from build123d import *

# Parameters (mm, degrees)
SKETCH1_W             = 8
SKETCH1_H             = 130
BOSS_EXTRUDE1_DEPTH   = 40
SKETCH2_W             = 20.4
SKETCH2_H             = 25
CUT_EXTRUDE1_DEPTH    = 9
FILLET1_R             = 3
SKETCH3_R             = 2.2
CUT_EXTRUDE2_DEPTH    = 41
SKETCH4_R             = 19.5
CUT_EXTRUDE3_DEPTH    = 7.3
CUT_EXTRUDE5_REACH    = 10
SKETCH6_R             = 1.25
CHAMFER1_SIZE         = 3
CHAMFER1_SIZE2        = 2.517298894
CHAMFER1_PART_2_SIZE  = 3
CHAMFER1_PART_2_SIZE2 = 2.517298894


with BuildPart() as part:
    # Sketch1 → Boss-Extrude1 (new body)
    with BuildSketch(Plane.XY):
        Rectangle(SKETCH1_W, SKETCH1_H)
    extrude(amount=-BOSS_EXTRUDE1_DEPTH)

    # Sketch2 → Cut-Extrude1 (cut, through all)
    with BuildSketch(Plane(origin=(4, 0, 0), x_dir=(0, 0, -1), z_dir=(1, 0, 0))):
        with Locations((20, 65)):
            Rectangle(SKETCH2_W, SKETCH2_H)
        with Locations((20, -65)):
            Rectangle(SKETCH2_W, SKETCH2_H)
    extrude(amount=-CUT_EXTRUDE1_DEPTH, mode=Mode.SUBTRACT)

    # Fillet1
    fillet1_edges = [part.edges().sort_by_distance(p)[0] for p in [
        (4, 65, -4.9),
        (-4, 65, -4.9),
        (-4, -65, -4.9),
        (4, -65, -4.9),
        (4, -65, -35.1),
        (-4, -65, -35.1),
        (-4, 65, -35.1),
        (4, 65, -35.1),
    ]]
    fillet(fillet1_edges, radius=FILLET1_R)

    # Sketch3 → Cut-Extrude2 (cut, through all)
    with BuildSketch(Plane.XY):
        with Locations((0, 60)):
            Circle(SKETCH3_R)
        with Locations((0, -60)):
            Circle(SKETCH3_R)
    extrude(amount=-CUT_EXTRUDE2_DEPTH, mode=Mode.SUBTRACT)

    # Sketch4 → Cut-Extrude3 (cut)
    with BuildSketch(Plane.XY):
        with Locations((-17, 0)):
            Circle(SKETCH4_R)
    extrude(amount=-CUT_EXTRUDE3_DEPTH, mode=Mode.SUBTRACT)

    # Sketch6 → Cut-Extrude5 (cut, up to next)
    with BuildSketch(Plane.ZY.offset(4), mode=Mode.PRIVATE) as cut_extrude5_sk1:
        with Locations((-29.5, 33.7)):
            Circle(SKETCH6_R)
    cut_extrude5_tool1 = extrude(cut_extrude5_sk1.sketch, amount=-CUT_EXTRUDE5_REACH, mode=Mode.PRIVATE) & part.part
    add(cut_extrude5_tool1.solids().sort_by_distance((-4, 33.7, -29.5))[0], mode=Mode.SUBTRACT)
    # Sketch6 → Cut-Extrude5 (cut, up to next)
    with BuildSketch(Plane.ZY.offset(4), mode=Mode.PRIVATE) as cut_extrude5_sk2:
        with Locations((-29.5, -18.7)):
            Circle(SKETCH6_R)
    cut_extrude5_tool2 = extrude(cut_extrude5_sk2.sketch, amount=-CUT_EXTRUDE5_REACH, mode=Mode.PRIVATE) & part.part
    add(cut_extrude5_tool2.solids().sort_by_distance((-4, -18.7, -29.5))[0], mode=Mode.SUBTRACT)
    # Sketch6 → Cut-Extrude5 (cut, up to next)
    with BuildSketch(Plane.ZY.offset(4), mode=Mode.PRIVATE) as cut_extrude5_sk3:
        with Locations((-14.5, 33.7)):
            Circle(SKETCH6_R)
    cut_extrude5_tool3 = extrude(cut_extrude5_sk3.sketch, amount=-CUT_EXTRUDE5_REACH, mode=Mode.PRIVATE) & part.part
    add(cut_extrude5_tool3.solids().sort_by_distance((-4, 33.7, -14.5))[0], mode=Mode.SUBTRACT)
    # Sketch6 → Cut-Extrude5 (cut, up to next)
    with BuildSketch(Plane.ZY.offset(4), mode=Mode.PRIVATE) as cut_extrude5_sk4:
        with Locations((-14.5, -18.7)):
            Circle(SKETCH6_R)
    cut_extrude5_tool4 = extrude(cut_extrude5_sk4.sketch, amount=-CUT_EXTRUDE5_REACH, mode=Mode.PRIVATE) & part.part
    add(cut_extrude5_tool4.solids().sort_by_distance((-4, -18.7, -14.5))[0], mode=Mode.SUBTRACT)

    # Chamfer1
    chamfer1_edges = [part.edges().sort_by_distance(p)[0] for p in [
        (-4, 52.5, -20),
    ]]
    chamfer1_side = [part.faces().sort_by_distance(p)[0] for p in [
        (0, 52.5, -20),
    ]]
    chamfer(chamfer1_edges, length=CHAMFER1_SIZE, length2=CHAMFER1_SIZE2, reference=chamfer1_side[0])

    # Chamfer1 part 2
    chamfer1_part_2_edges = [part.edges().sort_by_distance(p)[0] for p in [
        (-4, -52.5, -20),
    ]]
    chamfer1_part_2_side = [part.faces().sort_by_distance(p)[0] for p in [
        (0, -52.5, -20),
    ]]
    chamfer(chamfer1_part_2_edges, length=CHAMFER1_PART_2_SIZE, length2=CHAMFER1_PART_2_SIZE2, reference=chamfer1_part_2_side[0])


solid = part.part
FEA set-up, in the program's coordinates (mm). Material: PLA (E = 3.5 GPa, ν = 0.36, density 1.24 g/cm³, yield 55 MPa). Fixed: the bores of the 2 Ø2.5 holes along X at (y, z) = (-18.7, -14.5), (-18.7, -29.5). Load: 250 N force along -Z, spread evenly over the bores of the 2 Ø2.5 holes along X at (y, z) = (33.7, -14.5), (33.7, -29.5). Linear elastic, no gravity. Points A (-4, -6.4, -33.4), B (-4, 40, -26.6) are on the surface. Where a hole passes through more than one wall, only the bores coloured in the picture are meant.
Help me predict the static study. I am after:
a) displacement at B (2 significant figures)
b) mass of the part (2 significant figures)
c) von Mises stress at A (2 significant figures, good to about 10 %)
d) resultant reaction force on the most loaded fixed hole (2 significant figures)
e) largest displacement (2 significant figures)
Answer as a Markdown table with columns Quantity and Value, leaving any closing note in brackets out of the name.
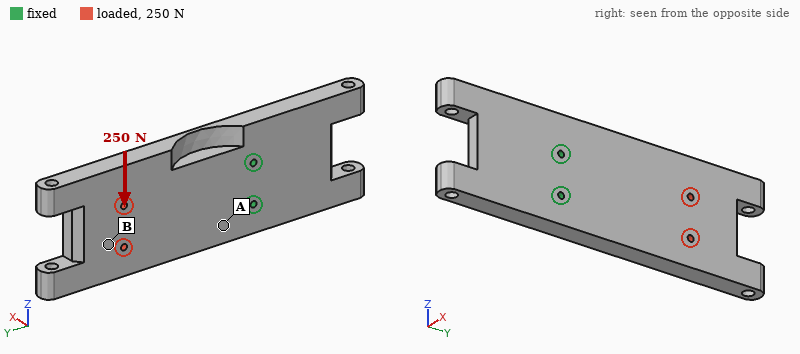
| Quantity | Value |
|---|---|
| displacement at B | 0.29 mm |
| mass of the part | 44 g |
| von Mises stress at A | 3.8 MPa |
| resultant reaction force on the most loaded fixed hole | 820 N |
| largest displacement | 0.43 mm |
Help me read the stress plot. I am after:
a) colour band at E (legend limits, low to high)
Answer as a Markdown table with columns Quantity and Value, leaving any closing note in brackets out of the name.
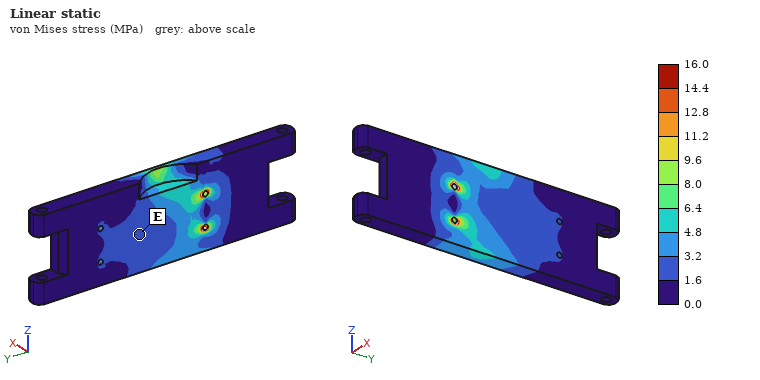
| Quantity | Value |
|---|---|
| colour band at E | 1.6 to 3.2 MPa |
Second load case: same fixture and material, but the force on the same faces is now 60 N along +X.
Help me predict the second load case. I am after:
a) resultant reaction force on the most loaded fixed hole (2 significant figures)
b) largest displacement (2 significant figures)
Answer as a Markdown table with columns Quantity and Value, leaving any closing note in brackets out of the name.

| Quantity | Value |
|---|---|
| resultant reaction force on the most loaded fixed hole | 31 N |
| largest displacement | 1.1 mm |
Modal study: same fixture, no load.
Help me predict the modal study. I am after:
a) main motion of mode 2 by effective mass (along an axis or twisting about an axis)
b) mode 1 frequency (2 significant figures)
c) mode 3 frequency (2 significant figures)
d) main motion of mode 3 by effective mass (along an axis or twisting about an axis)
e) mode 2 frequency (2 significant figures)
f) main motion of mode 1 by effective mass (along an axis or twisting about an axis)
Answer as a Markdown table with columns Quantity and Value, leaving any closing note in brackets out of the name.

| Quantity | Value |
|---|---|
| main motion of mode 2 by effective mass | along Z |
| mode 1 frequency | 330 Hz |
| mode 3 frequency | 1200 Hz |
| main motion of mode 3 by effective mass | twisting about Y |
| mode 2 frequency | 1000 Hz |
| main motion of mode 1 by effective mass | along X |
